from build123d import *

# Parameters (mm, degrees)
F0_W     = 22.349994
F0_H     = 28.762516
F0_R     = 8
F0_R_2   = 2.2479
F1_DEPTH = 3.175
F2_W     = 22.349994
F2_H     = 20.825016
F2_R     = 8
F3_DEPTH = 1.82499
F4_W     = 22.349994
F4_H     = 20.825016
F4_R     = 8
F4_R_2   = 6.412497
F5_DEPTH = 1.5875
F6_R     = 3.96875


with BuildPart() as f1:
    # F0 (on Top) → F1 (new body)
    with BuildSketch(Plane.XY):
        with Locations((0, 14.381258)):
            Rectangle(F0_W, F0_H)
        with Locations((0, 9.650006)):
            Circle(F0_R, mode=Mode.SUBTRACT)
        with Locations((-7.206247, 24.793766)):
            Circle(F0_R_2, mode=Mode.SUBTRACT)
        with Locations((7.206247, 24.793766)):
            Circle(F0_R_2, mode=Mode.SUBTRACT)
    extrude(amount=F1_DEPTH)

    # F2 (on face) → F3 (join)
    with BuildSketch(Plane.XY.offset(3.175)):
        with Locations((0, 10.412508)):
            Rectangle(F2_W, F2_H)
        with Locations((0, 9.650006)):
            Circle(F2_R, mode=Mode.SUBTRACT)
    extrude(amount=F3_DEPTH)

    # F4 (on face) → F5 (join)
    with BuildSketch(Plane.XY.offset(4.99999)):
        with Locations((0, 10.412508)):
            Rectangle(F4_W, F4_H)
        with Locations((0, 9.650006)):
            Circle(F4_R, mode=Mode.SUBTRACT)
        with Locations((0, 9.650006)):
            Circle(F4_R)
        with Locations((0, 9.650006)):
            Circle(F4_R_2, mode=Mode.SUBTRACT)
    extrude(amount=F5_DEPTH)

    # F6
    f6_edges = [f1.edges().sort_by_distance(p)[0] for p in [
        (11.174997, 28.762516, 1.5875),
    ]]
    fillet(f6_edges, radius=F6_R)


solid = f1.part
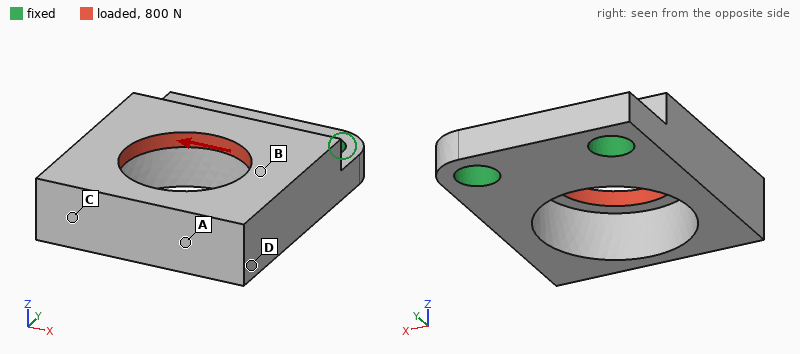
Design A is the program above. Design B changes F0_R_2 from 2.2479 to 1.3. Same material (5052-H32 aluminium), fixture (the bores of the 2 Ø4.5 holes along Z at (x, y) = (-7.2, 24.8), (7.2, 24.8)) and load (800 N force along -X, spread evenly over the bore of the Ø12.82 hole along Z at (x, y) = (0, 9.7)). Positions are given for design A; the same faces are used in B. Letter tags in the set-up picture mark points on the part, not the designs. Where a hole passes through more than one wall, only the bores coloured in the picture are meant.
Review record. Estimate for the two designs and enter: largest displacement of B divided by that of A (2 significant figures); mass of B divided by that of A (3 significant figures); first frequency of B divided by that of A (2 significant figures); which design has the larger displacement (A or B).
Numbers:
1.1
1.03
0.86
B
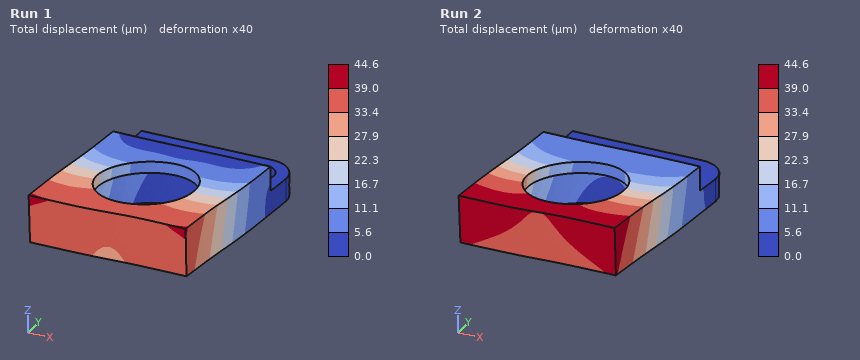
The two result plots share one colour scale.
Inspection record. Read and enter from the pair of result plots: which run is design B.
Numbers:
Run 2
